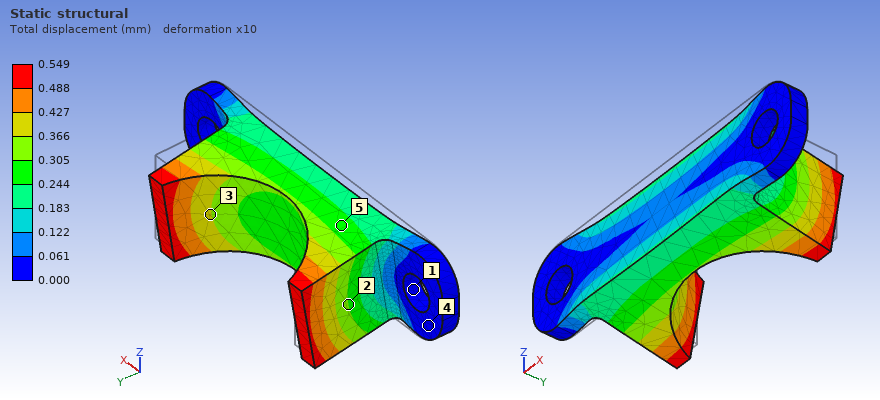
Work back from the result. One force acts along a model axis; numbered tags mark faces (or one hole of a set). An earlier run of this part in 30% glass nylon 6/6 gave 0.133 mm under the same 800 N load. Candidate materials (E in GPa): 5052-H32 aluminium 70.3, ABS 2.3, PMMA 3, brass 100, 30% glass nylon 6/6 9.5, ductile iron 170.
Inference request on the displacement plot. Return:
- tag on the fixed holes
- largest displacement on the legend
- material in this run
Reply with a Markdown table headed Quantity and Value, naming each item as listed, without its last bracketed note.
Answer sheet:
| Quantity | Value |
|---|---|
| tag on the fixed holes | 1 |
| largest displacement on the legend | 0.549 mm |
| material in this run | ABS |
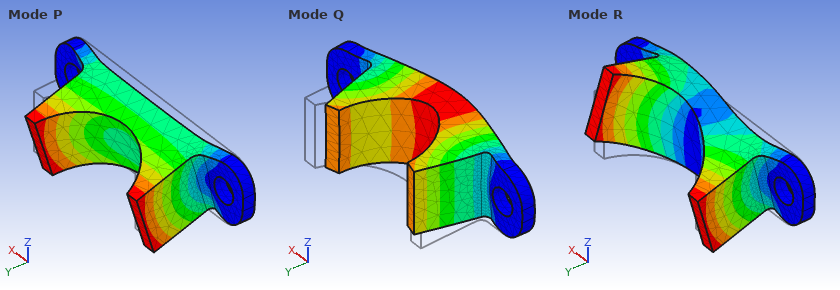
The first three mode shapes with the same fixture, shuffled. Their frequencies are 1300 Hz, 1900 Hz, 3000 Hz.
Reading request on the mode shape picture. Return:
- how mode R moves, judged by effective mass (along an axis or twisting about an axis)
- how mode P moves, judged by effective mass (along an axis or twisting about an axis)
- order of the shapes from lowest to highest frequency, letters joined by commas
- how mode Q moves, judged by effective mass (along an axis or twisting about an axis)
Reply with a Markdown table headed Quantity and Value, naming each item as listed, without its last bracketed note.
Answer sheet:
| Quantity | Value |
|---|---|
| how mode R moves, judged by effective mass | twisting about Y |
| how mode P moves, judged by effective mass | along Z |
| order of the shapes from lowest to highest frequency, letters joined by commas | P, Q, R |
| how mode Q moves, judged by effective mass | along Y |
